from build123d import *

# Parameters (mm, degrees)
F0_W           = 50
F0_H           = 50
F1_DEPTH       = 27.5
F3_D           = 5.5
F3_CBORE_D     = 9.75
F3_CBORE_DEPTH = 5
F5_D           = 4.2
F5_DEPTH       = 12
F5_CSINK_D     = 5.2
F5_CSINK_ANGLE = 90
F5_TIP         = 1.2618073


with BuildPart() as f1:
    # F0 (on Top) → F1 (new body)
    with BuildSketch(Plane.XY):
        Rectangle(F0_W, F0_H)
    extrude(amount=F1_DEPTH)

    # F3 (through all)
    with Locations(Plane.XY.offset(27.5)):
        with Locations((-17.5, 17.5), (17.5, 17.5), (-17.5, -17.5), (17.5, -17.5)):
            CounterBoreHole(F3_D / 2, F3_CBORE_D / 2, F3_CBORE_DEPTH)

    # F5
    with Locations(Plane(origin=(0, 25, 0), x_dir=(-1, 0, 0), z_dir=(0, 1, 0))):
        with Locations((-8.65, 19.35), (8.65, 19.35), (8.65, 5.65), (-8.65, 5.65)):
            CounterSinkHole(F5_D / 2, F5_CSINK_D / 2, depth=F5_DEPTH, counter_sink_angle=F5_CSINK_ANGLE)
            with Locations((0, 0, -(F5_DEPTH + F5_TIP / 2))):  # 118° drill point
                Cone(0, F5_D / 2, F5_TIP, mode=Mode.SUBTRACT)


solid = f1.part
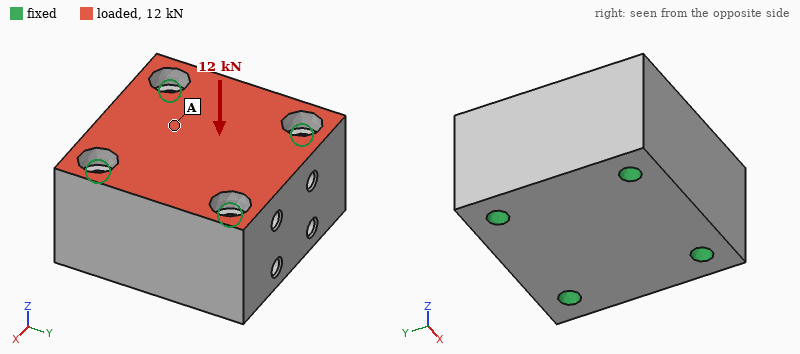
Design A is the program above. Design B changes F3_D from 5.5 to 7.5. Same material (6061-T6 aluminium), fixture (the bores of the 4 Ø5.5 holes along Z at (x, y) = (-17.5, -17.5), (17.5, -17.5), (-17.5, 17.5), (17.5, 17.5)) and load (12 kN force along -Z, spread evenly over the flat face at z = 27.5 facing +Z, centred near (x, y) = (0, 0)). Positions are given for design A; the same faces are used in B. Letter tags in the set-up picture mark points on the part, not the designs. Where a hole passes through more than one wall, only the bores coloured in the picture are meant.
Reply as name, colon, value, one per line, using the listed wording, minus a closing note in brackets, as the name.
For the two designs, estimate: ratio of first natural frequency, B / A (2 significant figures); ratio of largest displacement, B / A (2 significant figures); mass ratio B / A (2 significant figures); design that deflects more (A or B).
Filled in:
ratio of first natural frequency, B / A: 1.1
ratio of largest displacement, B / A: 0.87
mass ratio B / A: 0.97
design that deflects more: A
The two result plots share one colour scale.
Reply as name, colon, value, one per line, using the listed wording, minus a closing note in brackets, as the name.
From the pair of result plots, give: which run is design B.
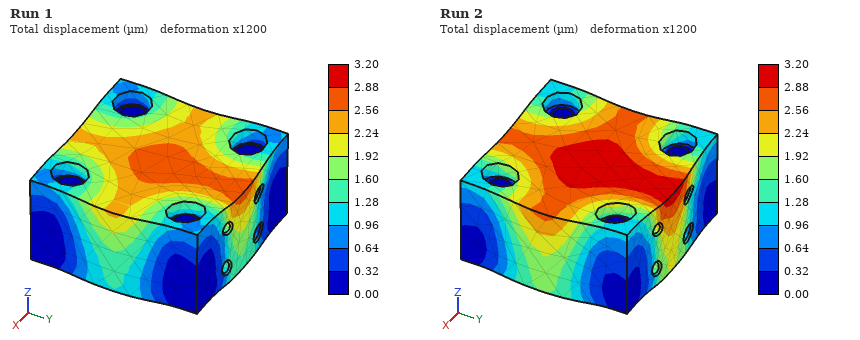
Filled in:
which run is design B: Run 1
